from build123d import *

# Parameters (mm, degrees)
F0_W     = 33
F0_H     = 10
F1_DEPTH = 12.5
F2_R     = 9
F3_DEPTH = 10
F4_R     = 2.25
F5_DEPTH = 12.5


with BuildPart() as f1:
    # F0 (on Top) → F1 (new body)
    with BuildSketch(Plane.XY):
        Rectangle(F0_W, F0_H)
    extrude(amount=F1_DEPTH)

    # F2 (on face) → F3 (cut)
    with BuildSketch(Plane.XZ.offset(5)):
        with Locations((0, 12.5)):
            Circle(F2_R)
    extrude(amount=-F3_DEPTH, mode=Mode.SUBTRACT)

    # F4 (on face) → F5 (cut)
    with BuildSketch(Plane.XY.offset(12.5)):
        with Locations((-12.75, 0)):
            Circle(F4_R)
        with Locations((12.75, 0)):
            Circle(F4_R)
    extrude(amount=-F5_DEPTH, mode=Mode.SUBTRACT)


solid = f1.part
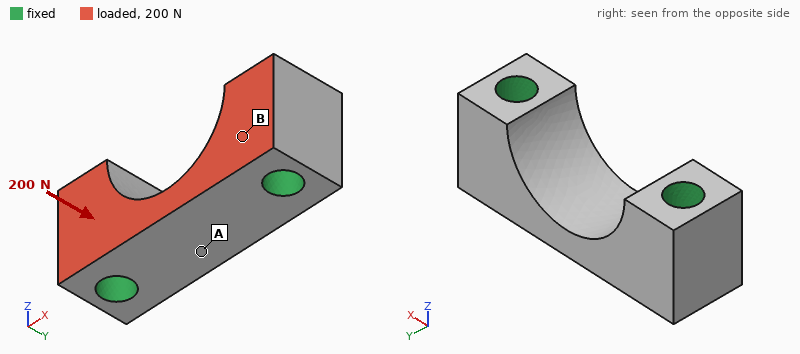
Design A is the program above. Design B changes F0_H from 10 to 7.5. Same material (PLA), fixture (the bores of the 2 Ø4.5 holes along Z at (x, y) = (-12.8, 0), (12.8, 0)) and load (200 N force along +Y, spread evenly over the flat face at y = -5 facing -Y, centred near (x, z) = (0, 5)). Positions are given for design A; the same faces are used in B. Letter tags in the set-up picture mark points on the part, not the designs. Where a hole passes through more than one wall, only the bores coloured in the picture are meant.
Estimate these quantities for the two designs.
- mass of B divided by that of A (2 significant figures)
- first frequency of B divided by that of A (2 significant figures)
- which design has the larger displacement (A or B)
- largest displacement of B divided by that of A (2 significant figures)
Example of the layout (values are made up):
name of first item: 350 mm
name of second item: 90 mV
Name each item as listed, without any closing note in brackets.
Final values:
mass of B divided by that of A: 0.71
first frequency of B divided by that of A: 0.97
which design has the larger displacement: B
largest displacement of B divided by that of A: 1.4
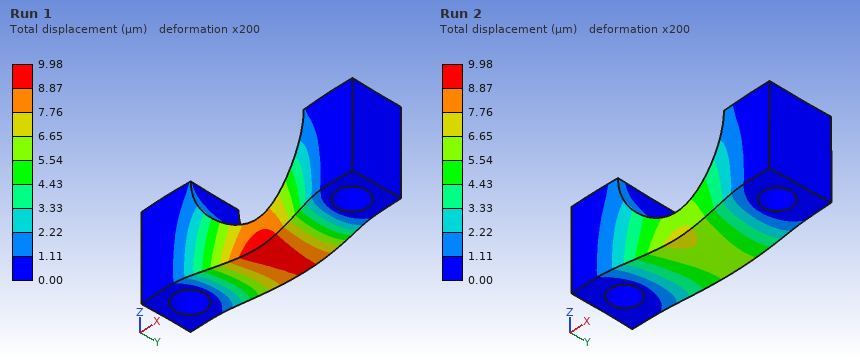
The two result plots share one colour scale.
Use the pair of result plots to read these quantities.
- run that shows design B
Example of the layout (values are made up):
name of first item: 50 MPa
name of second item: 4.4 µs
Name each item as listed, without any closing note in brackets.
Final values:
run that shows design B: Run 1
